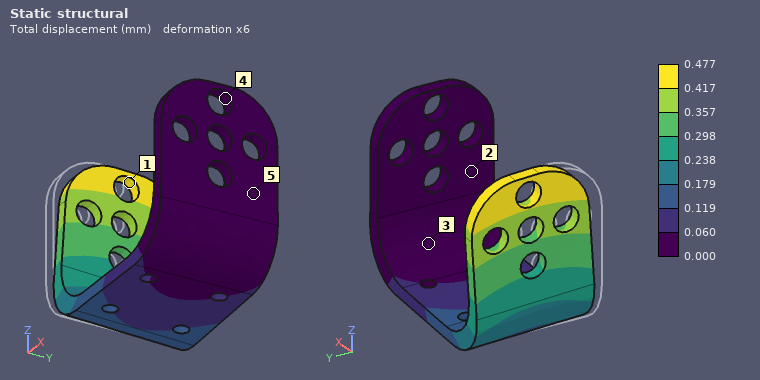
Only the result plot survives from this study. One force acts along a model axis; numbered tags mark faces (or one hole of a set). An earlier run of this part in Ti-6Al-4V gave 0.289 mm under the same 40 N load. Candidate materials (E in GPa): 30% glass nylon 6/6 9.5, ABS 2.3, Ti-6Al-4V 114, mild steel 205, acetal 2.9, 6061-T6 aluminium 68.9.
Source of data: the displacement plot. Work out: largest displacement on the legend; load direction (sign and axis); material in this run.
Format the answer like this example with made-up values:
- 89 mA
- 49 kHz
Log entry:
- 0.477 mm
- +Y
- 6061-T6 aluminium
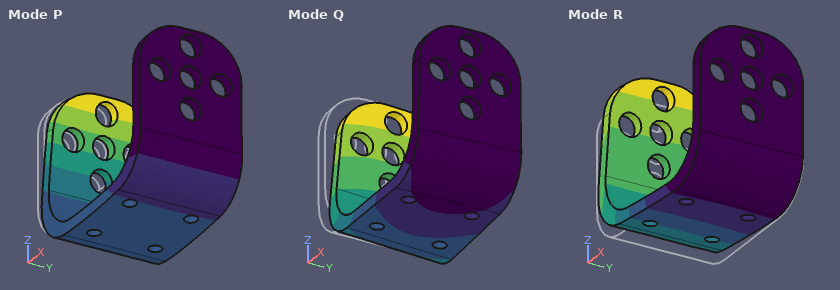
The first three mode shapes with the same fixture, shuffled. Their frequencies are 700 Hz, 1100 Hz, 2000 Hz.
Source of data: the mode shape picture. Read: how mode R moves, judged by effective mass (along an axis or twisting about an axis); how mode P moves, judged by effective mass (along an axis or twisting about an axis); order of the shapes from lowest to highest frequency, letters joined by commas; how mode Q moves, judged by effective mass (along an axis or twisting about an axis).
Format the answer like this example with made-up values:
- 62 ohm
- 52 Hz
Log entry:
- along Z
- along X
- R, Q, P
- along Y
